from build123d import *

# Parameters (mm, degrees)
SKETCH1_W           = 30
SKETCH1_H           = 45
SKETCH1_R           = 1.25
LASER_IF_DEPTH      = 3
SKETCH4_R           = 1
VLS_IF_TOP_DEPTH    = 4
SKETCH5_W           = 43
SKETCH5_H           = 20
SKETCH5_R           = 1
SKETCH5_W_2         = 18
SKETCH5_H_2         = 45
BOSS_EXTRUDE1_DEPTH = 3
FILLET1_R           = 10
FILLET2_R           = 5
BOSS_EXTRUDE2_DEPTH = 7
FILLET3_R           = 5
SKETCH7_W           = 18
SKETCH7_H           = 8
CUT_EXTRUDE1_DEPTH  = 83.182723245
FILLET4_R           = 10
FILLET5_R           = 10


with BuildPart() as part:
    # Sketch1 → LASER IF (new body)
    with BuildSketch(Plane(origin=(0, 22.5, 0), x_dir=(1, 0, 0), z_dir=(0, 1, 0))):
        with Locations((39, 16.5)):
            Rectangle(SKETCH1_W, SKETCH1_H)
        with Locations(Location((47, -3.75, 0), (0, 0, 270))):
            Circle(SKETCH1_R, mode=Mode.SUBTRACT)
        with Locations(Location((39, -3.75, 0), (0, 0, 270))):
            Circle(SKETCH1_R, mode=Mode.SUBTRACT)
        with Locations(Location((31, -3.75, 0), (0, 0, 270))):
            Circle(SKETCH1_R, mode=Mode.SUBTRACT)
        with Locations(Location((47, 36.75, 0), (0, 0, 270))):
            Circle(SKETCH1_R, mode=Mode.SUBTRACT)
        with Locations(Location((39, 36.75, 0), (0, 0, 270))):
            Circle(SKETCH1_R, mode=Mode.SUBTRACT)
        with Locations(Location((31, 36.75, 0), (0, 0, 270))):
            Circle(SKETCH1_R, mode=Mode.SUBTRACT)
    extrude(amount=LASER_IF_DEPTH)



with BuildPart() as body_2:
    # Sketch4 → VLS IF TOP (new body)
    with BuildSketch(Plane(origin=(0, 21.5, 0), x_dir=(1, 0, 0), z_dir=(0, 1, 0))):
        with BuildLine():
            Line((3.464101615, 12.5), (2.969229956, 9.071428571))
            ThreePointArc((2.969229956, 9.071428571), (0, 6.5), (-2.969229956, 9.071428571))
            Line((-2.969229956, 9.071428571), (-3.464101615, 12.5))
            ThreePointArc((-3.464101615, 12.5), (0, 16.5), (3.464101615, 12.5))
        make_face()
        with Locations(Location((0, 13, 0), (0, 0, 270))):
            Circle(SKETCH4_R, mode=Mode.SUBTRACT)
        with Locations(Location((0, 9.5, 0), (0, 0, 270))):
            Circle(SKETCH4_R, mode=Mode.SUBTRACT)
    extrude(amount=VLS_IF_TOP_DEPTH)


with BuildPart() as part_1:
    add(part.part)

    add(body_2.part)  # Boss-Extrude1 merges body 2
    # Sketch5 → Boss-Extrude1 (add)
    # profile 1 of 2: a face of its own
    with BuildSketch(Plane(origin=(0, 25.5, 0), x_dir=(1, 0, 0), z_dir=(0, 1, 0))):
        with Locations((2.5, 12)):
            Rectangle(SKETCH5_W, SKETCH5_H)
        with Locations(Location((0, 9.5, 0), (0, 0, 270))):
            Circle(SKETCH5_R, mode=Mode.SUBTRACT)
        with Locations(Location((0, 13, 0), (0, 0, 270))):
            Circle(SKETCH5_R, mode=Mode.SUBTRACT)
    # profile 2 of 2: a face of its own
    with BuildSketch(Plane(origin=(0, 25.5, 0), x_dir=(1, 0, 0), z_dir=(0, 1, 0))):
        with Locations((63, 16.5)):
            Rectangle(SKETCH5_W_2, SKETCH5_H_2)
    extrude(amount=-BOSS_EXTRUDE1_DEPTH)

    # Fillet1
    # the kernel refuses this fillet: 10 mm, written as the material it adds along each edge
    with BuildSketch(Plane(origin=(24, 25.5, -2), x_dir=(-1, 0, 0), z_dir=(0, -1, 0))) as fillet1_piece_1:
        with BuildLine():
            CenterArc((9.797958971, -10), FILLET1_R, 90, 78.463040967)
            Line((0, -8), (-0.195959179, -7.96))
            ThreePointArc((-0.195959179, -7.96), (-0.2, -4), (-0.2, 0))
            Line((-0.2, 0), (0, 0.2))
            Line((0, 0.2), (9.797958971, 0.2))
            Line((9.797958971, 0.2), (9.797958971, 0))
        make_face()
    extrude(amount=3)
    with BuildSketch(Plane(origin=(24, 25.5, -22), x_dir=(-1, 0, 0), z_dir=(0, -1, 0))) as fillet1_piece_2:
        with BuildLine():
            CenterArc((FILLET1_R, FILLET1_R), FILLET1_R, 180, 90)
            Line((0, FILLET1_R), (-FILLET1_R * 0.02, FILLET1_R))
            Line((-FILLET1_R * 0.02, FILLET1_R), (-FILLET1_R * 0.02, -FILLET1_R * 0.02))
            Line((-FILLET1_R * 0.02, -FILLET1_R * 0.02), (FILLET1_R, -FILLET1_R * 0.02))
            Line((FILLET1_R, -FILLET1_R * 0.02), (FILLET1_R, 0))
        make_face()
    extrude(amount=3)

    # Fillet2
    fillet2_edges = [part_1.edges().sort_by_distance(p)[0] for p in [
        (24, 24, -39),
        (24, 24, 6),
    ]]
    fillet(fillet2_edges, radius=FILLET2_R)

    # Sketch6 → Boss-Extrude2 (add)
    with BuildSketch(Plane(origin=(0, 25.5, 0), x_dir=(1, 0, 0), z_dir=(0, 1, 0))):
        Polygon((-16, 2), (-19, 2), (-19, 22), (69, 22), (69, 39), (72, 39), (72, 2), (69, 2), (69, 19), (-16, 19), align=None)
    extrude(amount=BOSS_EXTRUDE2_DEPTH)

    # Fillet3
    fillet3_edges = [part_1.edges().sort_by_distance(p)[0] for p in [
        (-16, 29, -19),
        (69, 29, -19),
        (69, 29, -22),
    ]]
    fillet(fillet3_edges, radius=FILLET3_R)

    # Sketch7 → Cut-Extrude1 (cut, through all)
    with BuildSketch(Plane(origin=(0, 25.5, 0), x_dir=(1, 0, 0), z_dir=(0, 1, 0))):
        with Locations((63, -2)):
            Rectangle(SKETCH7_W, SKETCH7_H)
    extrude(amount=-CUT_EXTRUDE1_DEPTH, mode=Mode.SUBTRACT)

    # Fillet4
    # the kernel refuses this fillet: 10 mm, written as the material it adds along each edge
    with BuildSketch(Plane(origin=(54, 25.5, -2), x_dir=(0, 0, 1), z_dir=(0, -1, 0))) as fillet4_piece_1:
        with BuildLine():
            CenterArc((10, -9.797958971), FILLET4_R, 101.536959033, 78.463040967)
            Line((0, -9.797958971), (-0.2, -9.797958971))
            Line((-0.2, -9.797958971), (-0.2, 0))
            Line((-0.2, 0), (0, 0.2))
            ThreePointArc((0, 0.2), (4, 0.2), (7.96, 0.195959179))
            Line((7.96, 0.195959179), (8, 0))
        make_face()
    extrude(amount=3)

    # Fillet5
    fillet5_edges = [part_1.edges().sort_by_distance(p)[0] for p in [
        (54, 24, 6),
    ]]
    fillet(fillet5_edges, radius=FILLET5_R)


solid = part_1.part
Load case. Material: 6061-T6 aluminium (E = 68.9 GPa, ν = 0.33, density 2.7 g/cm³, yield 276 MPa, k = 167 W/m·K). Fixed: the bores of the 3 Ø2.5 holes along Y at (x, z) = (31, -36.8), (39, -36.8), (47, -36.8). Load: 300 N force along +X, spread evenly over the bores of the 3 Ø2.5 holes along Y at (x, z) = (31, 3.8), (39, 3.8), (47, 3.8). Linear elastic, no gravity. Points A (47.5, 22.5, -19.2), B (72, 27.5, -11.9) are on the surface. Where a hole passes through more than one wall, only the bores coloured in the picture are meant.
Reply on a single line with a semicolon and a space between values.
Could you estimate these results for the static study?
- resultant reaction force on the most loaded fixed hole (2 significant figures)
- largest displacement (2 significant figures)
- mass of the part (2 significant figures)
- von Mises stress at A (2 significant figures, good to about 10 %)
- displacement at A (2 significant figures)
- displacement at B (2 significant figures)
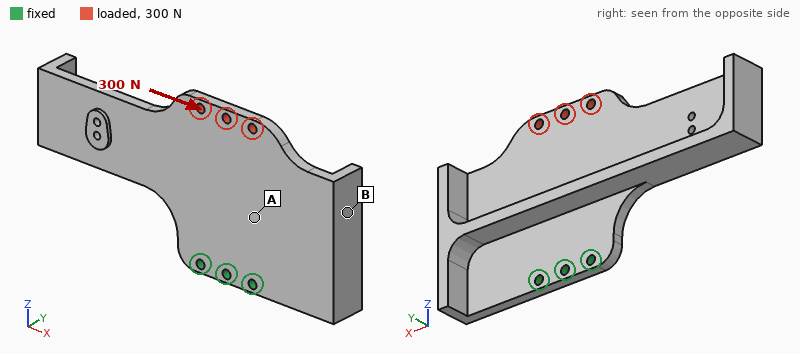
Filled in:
670 N; 43 µm; 32 g; 8.6 MPa; 11 µm; 25 µm
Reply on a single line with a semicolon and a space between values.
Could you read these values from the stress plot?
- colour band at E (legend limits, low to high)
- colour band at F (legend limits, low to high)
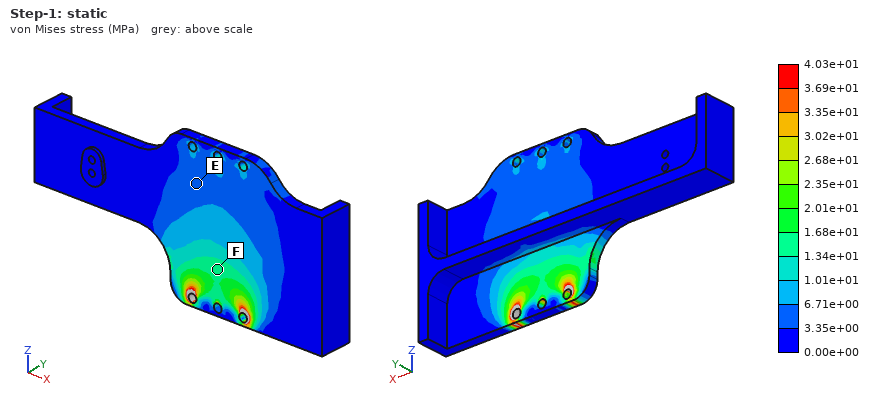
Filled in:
3.35e+00 to 6.71e+00 MPa; 1.34e+01 to 1.68e+01 MPa
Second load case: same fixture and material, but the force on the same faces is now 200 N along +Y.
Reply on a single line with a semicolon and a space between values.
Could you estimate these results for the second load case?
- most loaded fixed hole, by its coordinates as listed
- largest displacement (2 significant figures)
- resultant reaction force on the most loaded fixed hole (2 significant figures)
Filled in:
(39, -36.8); 0.73 mm; 130 N
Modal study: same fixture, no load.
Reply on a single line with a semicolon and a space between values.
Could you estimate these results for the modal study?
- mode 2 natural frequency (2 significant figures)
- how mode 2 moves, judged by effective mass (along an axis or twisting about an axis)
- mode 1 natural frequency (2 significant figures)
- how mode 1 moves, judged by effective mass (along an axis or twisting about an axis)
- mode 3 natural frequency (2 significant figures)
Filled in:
1200 Hz; along Y; 830 Hz; along Y; 3000 Hz
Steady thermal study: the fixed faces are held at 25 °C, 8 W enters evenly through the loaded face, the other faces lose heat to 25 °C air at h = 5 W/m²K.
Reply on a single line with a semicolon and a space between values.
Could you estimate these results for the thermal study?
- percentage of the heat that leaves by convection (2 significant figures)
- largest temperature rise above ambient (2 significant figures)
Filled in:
4.4 %; 18 K
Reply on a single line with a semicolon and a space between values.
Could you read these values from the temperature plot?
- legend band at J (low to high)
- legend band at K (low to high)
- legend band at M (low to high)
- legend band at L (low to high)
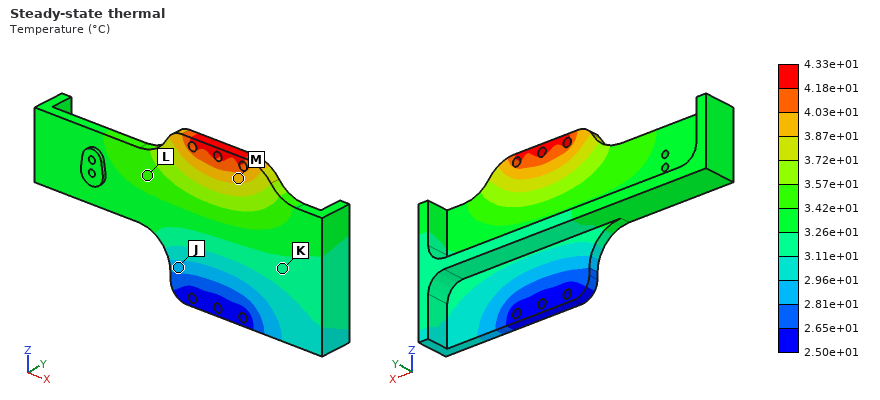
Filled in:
2.81e+01 to 2.96e+01 °C; 3.11e+01 to 3.26e+01 °C; 3.87e+01 to 4.03e+01 °C; 3.42e+01 to 3.57e+01 °C
